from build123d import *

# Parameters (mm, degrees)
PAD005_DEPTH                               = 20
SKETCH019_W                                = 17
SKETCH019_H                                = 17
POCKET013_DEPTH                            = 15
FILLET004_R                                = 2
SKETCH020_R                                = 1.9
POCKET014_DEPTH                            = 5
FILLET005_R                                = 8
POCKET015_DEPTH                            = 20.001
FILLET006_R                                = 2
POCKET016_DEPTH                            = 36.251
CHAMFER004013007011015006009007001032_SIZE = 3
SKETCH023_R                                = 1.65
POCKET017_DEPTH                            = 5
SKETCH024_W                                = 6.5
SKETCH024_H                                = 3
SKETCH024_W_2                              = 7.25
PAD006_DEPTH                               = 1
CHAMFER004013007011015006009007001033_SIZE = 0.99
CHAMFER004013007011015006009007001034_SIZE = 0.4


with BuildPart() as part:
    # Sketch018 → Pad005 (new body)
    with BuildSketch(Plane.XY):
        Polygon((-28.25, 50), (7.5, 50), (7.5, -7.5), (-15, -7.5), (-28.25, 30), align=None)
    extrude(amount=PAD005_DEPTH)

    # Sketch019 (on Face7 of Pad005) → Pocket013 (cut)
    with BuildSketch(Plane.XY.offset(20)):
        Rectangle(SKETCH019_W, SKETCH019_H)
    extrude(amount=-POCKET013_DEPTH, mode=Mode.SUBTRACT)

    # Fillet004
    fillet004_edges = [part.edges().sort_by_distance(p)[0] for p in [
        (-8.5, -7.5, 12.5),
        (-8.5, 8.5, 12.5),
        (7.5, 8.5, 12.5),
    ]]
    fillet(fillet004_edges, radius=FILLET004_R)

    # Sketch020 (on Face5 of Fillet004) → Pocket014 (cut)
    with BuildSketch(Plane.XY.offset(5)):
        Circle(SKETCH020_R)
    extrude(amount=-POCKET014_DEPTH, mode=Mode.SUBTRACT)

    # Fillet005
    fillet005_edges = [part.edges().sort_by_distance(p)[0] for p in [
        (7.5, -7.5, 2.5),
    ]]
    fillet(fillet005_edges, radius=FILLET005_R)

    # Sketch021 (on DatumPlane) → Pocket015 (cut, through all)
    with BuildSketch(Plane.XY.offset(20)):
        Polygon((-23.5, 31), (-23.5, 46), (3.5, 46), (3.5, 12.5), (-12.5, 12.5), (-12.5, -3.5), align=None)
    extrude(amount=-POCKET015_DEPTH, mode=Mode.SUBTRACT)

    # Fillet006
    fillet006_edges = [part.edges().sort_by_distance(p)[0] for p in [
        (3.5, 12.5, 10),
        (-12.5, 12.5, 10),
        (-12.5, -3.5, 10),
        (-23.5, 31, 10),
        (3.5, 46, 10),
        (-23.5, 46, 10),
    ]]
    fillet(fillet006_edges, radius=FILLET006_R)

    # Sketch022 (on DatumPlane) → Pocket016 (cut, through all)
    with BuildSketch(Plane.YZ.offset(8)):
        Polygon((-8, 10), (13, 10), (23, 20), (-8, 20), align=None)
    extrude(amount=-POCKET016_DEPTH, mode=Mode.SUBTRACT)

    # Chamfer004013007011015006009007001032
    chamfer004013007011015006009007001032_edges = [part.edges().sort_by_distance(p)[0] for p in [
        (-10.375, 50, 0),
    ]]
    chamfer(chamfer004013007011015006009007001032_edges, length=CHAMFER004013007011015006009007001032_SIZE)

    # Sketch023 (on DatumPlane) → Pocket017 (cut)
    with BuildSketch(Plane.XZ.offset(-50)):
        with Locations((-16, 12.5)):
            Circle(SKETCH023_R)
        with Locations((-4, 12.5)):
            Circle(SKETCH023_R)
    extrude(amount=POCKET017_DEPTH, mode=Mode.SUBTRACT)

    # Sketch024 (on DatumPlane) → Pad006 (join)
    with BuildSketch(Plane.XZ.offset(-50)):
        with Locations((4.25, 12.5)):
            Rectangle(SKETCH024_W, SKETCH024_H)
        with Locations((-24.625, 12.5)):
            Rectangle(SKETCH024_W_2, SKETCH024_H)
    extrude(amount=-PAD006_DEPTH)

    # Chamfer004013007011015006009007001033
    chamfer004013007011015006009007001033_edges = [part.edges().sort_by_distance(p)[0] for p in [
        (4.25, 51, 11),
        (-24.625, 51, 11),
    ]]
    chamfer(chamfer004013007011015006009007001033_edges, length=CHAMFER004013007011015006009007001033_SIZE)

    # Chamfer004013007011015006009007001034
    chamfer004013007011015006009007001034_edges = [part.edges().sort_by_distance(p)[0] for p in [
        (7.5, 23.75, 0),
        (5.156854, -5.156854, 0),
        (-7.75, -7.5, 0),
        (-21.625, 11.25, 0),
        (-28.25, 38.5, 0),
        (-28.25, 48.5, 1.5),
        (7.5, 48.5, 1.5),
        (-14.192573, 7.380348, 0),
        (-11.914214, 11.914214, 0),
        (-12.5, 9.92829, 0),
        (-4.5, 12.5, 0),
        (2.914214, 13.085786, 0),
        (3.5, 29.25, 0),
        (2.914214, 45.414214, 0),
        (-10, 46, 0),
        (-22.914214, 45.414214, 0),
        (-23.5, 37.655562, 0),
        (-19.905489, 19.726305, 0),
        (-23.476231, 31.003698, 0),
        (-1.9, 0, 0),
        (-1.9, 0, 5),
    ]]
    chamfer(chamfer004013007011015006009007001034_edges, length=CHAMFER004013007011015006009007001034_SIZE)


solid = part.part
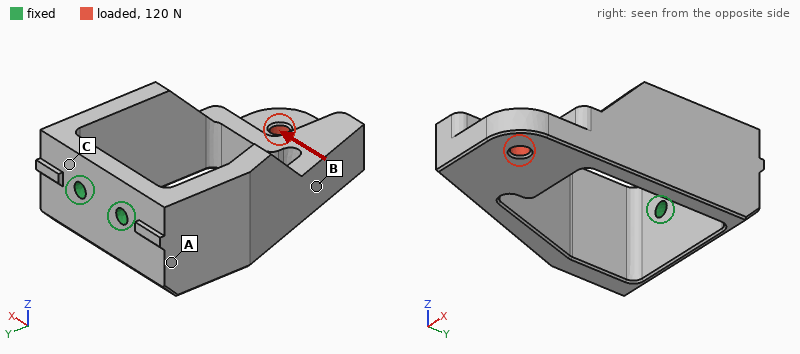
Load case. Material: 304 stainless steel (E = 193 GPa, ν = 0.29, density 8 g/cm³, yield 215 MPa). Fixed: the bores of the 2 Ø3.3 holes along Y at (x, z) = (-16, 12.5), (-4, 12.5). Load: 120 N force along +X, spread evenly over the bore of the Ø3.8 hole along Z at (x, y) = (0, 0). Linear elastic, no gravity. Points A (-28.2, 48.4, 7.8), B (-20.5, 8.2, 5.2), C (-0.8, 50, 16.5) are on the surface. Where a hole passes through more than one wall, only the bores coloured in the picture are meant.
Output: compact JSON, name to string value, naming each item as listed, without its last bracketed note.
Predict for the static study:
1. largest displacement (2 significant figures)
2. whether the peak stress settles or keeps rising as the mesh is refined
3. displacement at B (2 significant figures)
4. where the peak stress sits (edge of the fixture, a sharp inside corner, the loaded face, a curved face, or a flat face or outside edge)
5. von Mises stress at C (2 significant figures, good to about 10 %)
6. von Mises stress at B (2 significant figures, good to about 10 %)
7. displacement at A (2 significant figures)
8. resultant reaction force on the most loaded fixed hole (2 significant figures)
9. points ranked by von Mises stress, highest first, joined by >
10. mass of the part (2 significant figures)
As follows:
{"largest displacement": "36 µm", "whether the peak stress settles or keeps rising as the mesh is refined": "keeps rising", "displacement at B": "33 µm", "where the peak stress sits": "edge of the fixture", "von Mises stress at C": "30 MPa", "von Mises stress at B": "17 MPa", "displacement at A": "6.8 µm", "resultant reaction force on the most loaded fixed hole": "260 N", "points ranked by von Mises stress, highest first, joined by >": "C > B > A", "mass of the part": "93 g"}
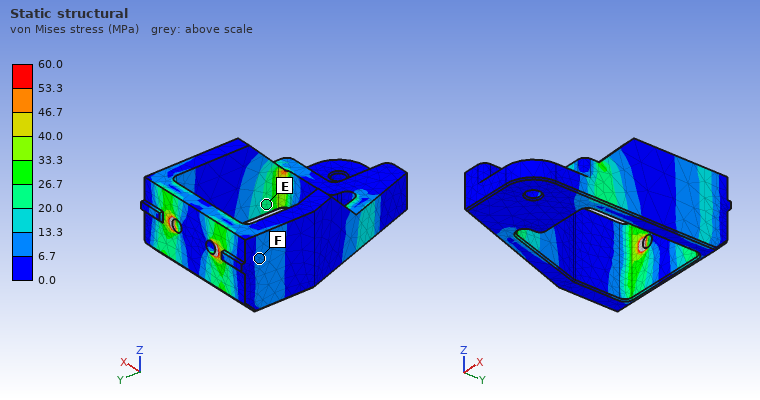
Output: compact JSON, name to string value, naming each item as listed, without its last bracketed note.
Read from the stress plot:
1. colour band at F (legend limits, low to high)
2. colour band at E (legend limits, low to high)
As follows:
{"colour band at F": "6.7 to 13.3 MPa", "colour band at E": "20.0 to 26.7 MPa"}
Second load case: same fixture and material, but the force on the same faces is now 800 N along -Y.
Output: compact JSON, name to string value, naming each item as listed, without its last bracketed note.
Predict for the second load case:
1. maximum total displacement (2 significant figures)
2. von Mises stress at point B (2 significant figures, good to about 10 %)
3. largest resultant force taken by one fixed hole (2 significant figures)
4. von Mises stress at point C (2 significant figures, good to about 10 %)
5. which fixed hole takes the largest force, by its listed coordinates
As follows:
{"maximum total displacement": "82 µm", "von Mises stress at point B": "22 MPa", "largest resultant force taken by one fixed hole": "770 N", "von Mises stress at point C": "64 MPa", "which fixed hole takes the largest force, by its listed coordinates": "(-4, 12.5)"}
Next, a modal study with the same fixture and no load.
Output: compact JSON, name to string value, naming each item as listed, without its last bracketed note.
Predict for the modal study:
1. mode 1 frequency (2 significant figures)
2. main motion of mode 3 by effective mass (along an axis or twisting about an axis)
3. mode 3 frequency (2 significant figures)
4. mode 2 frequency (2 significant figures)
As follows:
{"mode 1 frequency": "1400 Hz", "main motion of mode 3 by effective mass": "twisting about Y", "mode 3 frequency": "4400 Hz", "mode 2 frequency": "1500 Hz"}
